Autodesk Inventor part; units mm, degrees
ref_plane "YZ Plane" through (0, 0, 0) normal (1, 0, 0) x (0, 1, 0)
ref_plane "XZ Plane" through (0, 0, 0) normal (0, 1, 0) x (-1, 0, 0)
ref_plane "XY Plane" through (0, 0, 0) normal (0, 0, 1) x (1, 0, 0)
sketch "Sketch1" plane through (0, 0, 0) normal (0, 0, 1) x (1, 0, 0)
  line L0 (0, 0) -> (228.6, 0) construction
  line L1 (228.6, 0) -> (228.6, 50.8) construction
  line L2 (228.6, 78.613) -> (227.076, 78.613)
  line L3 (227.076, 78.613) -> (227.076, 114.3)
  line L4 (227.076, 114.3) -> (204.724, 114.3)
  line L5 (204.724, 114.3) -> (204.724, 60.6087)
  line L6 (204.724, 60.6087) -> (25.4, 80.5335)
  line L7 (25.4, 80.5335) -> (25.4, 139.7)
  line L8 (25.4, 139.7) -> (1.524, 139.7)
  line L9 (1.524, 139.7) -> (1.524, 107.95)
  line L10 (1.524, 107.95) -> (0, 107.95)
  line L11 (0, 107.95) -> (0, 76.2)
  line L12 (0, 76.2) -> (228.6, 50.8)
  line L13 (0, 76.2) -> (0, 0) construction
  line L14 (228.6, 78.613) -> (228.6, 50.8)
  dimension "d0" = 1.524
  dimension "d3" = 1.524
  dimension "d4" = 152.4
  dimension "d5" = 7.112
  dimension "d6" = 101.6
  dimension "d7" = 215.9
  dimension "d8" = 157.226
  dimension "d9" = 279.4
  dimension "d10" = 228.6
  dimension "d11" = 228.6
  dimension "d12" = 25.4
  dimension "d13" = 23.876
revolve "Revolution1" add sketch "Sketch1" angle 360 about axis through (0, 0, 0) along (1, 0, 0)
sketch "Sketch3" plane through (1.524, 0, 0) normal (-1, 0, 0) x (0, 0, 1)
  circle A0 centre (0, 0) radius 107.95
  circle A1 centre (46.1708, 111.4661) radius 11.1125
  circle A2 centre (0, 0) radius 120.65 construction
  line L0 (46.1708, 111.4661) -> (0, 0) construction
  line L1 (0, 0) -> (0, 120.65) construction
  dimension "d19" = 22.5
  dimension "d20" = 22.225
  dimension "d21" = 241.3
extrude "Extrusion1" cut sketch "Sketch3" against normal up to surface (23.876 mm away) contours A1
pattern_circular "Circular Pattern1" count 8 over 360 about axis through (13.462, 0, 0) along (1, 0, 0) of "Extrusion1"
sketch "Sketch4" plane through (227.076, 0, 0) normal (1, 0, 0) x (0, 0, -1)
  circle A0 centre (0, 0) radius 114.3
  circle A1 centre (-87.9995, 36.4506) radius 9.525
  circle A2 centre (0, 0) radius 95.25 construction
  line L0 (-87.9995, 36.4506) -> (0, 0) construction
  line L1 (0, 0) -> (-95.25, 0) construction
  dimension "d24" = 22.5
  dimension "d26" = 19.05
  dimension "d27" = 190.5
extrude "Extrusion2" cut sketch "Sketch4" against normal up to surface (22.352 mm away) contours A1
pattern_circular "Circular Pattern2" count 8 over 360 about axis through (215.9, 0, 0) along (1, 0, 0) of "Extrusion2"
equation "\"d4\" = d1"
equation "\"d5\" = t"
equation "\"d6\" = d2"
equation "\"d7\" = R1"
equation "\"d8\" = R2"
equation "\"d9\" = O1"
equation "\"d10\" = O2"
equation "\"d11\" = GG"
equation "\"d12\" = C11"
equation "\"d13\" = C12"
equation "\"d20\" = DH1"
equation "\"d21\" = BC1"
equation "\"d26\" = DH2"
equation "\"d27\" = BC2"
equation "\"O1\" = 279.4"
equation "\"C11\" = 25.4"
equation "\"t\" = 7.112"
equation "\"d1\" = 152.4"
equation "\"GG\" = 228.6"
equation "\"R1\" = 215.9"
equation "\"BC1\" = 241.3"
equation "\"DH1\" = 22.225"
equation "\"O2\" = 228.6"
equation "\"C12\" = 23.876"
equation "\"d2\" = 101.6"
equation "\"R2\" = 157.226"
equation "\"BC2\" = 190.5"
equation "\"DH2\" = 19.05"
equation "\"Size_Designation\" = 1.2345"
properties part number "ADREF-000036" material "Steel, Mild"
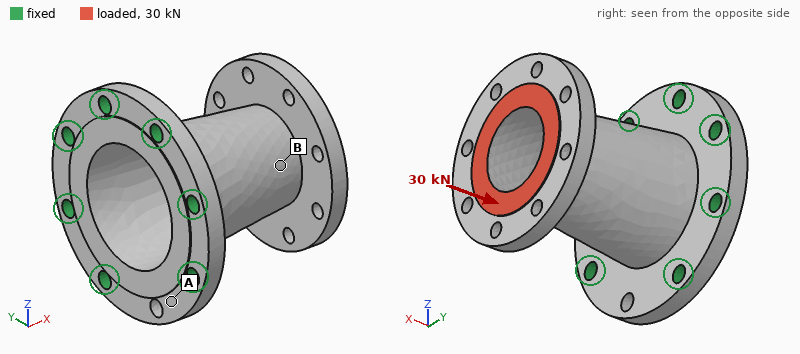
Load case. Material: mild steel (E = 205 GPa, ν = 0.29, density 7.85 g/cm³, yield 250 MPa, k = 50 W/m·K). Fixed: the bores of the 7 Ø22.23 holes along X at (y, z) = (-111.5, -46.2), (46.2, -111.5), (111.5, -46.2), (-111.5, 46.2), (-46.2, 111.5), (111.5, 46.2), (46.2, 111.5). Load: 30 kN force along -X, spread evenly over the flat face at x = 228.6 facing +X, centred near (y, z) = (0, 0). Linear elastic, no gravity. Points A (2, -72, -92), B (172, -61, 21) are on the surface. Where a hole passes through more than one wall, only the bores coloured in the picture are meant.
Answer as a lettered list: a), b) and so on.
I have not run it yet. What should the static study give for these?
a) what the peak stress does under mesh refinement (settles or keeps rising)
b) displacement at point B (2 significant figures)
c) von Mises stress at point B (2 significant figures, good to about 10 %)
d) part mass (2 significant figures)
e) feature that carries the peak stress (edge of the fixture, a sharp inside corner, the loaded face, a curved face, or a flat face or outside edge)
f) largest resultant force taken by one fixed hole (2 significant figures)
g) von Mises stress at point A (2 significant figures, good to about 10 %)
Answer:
a) keeps rising
b) 13 µm
c) 9.1 MPa
d) 18 kg
e) edge of the fixture
f) 5.8 kN
g) 3.7 MPa
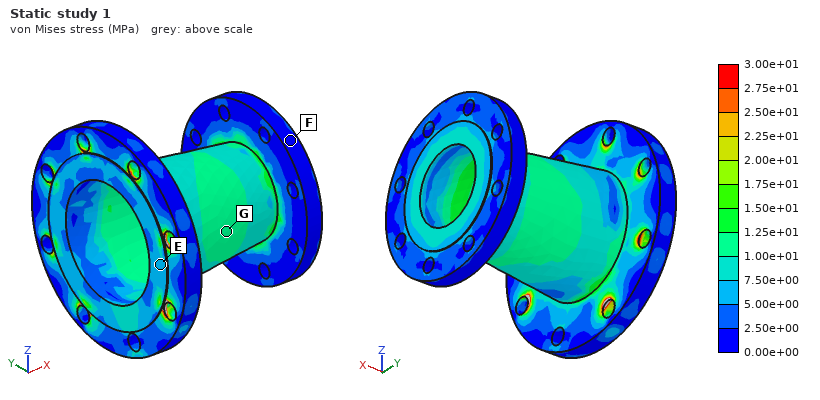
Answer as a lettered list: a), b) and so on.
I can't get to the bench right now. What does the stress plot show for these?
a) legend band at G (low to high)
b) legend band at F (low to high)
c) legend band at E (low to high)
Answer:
a) 1.00e+01 to 1.25e+01 MPa
b) 0.00e+00 to 2.50e+00 MPa
c) 5.00e+00 to 7.50e+00 MPa
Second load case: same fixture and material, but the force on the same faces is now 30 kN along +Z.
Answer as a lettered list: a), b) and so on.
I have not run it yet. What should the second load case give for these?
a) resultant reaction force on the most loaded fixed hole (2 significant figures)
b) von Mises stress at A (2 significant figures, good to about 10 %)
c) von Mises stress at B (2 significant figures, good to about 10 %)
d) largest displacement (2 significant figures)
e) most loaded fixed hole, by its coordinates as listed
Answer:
a) 26 kN
b) 14 MPa
c) 32 MPa
d) 0.19 mm
e) (46.2, -111.5)
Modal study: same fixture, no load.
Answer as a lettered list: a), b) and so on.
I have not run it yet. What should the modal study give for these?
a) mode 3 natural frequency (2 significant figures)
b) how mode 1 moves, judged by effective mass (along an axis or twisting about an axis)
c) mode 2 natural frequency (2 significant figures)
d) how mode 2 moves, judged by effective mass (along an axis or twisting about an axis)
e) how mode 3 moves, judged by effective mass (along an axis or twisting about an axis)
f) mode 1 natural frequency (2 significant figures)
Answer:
a) 1700 Hz
b) along Z
c) 930 Hz
d) along Y
e) twisting about X
f) 870 Hz
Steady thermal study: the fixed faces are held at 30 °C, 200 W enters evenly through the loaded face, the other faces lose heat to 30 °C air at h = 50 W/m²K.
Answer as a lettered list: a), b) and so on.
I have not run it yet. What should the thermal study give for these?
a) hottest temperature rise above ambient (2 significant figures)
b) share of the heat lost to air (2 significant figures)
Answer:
a) 39 K
b) 97 %
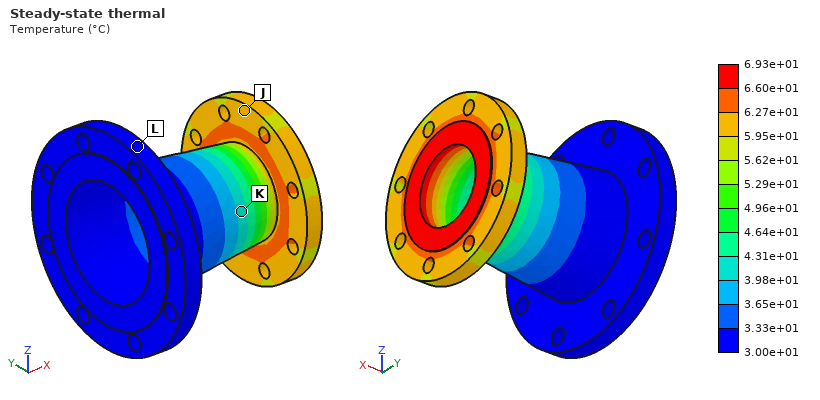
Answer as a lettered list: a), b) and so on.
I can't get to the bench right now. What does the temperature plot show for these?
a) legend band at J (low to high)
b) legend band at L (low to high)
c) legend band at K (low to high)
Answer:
a) 5.95e+01 to 6.27e+01 °C
b) 3.00e+01 to 3.33e+01 °C
c) 3.98e+01 to 4.31e+01 °C
